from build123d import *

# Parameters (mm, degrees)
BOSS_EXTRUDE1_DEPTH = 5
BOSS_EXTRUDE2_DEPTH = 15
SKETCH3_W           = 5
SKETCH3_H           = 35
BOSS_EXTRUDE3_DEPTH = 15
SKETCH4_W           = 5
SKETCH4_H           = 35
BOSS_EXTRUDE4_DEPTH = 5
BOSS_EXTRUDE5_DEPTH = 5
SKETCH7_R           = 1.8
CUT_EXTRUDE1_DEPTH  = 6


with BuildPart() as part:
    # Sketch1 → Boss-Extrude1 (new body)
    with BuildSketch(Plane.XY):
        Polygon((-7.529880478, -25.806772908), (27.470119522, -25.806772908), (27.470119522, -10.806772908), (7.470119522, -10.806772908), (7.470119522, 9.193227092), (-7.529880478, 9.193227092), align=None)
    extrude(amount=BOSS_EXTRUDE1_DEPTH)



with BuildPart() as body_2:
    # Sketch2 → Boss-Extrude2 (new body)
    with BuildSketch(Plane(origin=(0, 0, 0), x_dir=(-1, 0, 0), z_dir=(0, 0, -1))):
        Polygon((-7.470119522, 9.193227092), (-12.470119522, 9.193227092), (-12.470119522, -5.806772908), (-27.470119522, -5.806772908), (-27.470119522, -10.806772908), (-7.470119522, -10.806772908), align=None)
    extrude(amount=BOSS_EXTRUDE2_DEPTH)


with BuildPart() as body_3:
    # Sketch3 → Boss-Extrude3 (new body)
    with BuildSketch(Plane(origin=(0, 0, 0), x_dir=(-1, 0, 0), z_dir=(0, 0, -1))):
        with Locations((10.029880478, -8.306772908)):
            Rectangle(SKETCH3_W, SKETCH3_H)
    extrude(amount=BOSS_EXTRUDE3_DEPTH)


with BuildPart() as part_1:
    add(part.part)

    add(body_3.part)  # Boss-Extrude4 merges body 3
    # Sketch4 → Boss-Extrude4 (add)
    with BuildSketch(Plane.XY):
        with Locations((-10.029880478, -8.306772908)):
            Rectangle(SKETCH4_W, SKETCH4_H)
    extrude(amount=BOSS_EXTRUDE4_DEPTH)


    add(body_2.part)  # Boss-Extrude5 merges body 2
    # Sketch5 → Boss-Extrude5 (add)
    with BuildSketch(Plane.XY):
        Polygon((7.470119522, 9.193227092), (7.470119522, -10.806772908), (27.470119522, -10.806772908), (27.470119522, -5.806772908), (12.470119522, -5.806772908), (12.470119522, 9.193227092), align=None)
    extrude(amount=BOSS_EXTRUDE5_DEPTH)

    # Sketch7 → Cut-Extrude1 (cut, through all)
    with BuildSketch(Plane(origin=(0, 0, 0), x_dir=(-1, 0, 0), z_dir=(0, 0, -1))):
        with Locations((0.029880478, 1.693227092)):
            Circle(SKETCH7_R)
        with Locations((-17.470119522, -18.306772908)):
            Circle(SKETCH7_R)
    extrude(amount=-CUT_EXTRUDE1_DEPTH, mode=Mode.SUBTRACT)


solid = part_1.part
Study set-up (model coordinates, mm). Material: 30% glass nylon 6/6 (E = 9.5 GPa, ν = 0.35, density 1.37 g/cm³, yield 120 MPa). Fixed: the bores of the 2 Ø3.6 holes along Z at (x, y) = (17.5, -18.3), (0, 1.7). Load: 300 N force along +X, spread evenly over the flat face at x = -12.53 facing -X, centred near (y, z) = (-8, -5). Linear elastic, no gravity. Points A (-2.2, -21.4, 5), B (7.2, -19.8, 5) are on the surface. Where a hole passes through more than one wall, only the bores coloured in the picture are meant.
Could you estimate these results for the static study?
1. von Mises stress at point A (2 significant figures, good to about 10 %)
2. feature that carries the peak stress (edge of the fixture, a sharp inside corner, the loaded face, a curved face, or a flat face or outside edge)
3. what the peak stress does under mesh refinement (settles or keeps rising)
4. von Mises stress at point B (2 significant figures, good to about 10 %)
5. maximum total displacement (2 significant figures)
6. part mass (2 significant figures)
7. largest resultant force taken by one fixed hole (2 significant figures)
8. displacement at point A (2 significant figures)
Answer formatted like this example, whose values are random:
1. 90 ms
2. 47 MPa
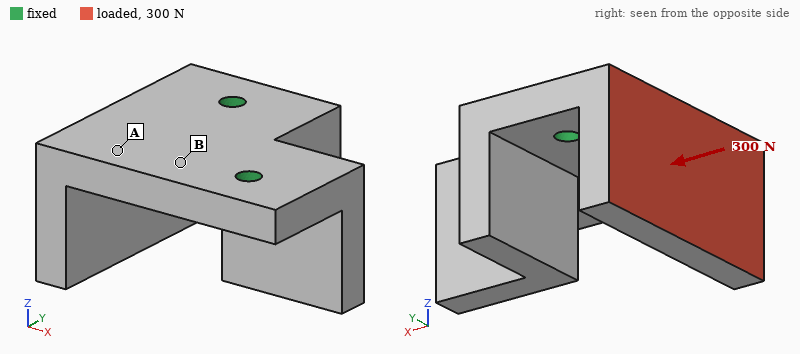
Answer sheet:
1. 9.0 MPa
2. edge of the fixture
3. keeps rising
4. 4.1 MPa
5. 0.22 mm
6. 15 g
7. 160 N
8. 0.035 mm
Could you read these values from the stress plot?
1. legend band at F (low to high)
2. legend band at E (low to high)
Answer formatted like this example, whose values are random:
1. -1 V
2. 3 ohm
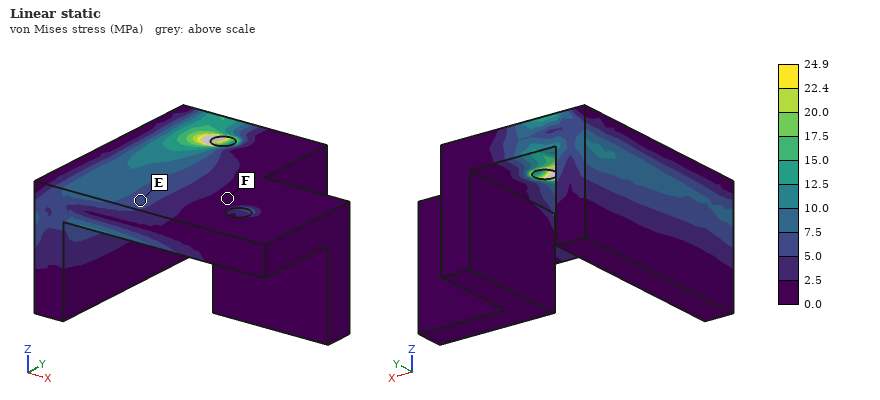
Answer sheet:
1. 0.0 to 2.5 MPa
2. 5.0 to 7.5 MPa
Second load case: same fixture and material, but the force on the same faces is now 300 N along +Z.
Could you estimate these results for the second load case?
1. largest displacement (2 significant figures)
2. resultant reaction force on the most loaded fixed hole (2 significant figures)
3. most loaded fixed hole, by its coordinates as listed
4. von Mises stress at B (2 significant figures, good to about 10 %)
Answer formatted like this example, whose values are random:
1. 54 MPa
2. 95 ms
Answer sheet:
1. 0.37 mm
2. 290 N
3. (0, 1.7)
4. 14 MPa
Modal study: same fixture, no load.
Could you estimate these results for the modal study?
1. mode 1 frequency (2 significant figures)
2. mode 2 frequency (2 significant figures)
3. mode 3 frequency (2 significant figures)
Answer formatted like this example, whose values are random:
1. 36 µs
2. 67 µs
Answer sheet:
1. 2400 Hz
2. 4100 Hz
3. 4900 Hz
